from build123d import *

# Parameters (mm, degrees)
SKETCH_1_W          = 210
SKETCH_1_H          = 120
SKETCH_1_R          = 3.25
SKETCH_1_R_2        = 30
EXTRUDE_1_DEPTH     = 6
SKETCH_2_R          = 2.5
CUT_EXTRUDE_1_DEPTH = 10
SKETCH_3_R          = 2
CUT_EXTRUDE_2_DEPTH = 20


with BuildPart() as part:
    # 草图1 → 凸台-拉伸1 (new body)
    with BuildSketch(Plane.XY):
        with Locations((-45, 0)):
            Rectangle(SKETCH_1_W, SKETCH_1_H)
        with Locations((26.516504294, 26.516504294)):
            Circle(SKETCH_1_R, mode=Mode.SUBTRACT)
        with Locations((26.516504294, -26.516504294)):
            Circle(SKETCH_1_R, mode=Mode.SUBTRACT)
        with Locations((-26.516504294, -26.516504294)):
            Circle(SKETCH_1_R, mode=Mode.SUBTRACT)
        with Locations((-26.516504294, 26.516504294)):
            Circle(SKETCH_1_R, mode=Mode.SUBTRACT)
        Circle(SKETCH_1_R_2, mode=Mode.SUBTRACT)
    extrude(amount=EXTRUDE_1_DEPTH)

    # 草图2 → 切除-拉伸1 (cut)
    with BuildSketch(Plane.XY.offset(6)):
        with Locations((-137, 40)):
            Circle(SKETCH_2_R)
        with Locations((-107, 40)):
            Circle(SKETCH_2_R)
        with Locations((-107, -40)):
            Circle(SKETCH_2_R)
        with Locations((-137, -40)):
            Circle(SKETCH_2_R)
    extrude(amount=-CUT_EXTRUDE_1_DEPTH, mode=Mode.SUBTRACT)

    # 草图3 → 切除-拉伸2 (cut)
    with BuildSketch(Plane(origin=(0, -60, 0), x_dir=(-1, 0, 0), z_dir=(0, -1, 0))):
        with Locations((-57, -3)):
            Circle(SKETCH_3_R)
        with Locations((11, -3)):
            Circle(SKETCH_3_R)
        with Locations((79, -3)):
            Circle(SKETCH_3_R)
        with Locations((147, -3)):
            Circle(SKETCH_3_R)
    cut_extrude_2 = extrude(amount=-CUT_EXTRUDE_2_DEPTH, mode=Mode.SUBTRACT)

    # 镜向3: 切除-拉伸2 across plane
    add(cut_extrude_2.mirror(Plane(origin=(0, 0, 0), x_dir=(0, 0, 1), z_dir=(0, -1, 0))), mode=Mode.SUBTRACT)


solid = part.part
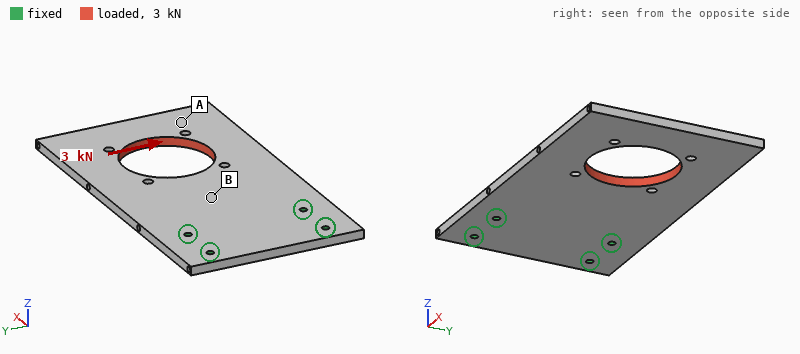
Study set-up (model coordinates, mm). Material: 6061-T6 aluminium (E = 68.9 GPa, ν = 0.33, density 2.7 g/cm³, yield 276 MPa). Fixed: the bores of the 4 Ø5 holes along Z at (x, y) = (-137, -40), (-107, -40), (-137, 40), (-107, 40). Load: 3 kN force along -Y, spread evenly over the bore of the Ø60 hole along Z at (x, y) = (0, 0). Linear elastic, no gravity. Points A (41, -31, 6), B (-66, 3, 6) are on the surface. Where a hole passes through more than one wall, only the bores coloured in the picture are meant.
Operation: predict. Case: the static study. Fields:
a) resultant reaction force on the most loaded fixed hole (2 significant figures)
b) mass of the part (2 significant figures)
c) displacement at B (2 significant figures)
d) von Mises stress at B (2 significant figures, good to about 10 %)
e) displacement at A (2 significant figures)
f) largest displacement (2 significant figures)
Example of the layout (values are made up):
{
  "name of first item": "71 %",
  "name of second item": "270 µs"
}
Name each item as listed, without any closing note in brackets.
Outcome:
{
  "resultant reaction force on the most loaded fixed hole": "3.3 kN",
  "mass of the part": "350 g",
  "displacement at B": "0.017 mm",
  "von Mises stress at B": "15 MPa",
  "displacement at A": "0.097 mm",
  "largest displacement": "0.11 mm"
}
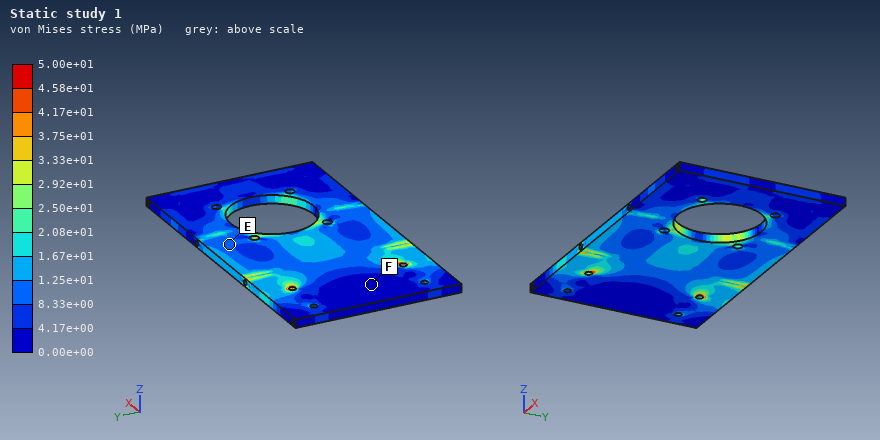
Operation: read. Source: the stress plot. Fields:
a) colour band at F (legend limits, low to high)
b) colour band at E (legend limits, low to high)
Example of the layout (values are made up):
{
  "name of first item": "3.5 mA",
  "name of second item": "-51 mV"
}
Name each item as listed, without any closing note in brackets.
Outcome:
{
  "colour band at F": "0.00e+00 to 4.17e+00 MPa",
  "colour band at E": "8.33e+00 to 1.25e+01 MPa"
}
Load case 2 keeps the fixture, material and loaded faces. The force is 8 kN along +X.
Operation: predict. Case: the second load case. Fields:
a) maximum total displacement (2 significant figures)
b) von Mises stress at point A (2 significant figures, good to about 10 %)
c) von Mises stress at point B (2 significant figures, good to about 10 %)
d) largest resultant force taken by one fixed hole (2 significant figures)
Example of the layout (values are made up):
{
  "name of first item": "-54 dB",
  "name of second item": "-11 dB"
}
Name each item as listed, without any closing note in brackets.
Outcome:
{
  "maximum total displacement": "45 µm",
  "von Mises stress at point A": "9.0 MPa",
  "von Mises stress at point B": "7.1 MPa",
  "largest resultant force taken by one fixed hole": "2.9 kN"
}
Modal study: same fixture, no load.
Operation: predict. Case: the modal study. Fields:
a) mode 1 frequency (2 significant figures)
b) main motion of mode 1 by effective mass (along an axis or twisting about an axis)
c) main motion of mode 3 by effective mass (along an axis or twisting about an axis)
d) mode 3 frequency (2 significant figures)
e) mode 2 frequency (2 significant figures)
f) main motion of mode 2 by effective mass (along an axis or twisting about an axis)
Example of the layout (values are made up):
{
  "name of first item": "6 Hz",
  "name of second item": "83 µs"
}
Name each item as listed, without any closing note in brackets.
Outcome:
{
  "mode 1 frequency": "180 Hz",
  "main motion of mode 1 by effective mass": "along Z",
  "main motion of mode 3 by effective mass": "along Z",
  "mode 3 frequency": "960 Hz",
  "mode 2 frequency": "510 Hz",
  "main motion of mode 2 by effective mass": "twisting about X"
}
